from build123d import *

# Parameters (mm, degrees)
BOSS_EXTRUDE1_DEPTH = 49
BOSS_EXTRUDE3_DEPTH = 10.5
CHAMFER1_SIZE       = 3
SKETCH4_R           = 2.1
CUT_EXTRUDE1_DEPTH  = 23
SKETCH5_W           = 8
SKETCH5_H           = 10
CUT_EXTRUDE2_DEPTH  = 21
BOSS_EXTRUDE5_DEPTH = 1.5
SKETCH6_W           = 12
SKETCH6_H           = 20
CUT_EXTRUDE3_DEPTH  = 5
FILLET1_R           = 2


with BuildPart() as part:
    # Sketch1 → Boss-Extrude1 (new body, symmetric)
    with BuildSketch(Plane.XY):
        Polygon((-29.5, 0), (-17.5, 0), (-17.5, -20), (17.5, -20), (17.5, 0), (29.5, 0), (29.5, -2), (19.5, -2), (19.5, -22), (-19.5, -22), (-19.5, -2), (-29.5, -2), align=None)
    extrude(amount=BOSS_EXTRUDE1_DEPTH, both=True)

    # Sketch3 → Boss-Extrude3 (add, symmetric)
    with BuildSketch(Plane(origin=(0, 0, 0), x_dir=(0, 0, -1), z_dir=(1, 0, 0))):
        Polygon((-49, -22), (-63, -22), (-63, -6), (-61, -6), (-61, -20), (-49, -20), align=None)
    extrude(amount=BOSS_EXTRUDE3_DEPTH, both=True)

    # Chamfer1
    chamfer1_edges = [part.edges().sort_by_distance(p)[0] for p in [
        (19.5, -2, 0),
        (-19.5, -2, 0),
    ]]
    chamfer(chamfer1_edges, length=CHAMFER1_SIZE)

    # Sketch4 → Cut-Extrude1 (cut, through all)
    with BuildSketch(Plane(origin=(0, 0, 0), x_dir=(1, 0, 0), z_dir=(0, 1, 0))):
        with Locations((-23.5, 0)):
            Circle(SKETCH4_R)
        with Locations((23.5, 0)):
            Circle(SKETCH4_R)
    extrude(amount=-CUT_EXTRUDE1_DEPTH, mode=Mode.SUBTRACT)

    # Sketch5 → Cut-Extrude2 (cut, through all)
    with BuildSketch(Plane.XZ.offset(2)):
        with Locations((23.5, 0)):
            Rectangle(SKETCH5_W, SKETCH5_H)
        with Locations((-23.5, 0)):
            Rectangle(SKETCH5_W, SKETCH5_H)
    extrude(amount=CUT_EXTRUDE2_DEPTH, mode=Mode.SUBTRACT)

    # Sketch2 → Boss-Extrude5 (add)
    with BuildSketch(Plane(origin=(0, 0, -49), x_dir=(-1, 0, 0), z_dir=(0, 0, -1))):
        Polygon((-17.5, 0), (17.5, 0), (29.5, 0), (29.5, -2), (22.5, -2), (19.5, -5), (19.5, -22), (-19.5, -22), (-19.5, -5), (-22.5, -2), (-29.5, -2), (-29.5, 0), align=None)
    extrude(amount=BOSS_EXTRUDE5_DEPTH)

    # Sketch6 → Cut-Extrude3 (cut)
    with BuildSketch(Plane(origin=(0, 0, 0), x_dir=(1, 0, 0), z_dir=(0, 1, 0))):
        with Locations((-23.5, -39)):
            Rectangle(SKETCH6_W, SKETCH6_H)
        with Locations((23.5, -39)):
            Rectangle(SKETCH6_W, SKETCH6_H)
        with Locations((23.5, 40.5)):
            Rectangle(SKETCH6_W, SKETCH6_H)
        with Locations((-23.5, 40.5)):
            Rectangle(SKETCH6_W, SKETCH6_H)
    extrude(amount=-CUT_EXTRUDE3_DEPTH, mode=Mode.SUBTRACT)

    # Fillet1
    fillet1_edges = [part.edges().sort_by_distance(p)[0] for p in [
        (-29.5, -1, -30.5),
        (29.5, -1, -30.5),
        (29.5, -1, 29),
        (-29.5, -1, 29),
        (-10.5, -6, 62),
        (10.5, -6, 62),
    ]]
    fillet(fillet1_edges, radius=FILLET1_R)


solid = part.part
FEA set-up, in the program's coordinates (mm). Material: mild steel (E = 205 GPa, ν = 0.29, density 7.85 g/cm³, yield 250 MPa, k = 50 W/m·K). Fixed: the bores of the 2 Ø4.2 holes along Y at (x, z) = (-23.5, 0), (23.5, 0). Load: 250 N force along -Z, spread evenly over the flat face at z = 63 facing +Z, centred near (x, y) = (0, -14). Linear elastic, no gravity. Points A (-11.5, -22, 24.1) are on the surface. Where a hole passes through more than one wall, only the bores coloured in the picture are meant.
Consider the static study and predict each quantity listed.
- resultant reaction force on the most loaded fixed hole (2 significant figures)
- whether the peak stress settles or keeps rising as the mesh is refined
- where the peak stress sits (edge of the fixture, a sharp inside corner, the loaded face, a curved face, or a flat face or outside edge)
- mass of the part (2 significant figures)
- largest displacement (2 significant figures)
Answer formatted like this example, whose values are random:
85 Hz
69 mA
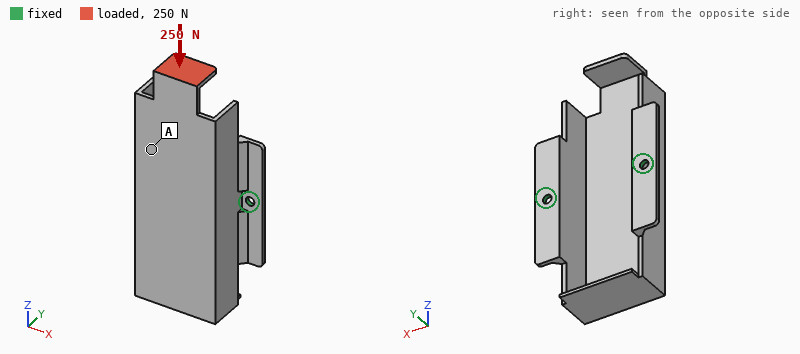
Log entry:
130 N
keeps rising
a sharp inside corner
160 g
0.22 mm
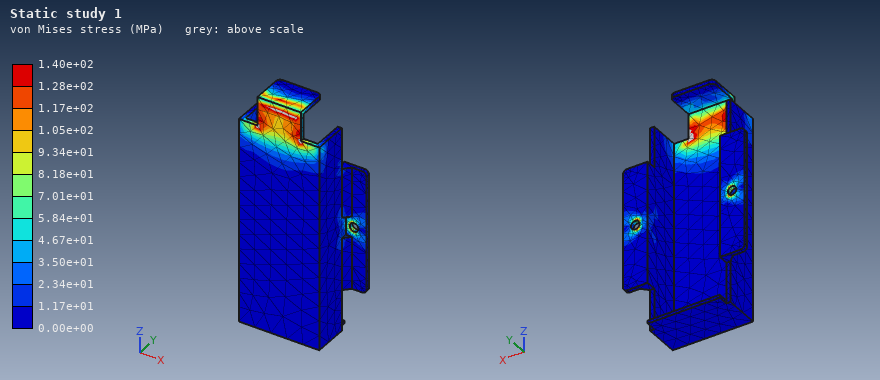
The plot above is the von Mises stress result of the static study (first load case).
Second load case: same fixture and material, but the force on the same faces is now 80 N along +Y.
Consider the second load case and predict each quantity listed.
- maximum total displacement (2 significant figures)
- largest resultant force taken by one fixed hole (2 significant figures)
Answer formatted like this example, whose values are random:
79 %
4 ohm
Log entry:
0.22 mm
43 N
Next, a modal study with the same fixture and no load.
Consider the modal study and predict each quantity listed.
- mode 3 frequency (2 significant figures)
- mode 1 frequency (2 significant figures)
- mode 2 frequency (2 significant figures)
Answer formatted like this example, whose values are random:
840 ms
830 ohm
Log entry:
1700 Hz
680 Hz
1400 Hz
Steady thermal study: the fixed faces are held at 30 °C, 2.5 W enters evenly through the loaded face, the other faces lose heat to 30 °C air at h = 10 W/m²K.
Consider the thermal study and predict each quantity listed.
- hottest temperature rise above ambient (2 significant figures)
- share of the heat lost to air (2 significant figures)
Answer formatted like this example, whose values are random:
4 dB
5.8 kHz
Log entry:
41 K
46 %
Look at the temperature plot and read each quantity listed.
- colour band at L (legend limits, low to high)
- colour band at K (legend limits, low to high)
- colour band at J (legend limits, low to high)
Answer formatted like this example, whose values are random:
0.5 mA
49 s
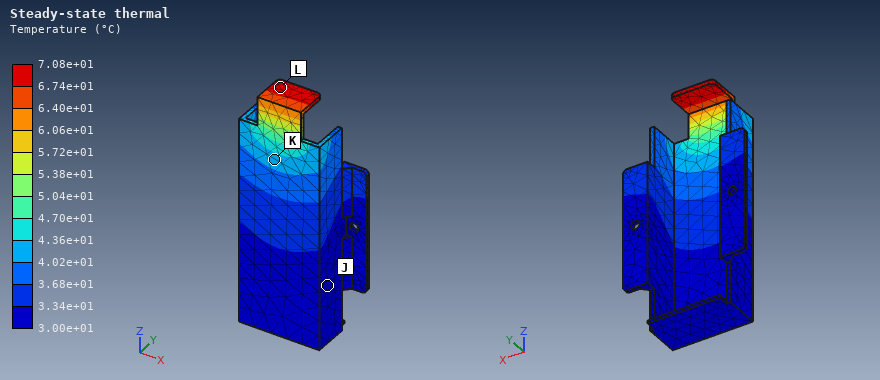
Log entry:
6.74e+01 to 7.08e+01 °C
4.02e+01 to 4.36e+01 °C
3.00e+01 to 3.34e+01 °C
